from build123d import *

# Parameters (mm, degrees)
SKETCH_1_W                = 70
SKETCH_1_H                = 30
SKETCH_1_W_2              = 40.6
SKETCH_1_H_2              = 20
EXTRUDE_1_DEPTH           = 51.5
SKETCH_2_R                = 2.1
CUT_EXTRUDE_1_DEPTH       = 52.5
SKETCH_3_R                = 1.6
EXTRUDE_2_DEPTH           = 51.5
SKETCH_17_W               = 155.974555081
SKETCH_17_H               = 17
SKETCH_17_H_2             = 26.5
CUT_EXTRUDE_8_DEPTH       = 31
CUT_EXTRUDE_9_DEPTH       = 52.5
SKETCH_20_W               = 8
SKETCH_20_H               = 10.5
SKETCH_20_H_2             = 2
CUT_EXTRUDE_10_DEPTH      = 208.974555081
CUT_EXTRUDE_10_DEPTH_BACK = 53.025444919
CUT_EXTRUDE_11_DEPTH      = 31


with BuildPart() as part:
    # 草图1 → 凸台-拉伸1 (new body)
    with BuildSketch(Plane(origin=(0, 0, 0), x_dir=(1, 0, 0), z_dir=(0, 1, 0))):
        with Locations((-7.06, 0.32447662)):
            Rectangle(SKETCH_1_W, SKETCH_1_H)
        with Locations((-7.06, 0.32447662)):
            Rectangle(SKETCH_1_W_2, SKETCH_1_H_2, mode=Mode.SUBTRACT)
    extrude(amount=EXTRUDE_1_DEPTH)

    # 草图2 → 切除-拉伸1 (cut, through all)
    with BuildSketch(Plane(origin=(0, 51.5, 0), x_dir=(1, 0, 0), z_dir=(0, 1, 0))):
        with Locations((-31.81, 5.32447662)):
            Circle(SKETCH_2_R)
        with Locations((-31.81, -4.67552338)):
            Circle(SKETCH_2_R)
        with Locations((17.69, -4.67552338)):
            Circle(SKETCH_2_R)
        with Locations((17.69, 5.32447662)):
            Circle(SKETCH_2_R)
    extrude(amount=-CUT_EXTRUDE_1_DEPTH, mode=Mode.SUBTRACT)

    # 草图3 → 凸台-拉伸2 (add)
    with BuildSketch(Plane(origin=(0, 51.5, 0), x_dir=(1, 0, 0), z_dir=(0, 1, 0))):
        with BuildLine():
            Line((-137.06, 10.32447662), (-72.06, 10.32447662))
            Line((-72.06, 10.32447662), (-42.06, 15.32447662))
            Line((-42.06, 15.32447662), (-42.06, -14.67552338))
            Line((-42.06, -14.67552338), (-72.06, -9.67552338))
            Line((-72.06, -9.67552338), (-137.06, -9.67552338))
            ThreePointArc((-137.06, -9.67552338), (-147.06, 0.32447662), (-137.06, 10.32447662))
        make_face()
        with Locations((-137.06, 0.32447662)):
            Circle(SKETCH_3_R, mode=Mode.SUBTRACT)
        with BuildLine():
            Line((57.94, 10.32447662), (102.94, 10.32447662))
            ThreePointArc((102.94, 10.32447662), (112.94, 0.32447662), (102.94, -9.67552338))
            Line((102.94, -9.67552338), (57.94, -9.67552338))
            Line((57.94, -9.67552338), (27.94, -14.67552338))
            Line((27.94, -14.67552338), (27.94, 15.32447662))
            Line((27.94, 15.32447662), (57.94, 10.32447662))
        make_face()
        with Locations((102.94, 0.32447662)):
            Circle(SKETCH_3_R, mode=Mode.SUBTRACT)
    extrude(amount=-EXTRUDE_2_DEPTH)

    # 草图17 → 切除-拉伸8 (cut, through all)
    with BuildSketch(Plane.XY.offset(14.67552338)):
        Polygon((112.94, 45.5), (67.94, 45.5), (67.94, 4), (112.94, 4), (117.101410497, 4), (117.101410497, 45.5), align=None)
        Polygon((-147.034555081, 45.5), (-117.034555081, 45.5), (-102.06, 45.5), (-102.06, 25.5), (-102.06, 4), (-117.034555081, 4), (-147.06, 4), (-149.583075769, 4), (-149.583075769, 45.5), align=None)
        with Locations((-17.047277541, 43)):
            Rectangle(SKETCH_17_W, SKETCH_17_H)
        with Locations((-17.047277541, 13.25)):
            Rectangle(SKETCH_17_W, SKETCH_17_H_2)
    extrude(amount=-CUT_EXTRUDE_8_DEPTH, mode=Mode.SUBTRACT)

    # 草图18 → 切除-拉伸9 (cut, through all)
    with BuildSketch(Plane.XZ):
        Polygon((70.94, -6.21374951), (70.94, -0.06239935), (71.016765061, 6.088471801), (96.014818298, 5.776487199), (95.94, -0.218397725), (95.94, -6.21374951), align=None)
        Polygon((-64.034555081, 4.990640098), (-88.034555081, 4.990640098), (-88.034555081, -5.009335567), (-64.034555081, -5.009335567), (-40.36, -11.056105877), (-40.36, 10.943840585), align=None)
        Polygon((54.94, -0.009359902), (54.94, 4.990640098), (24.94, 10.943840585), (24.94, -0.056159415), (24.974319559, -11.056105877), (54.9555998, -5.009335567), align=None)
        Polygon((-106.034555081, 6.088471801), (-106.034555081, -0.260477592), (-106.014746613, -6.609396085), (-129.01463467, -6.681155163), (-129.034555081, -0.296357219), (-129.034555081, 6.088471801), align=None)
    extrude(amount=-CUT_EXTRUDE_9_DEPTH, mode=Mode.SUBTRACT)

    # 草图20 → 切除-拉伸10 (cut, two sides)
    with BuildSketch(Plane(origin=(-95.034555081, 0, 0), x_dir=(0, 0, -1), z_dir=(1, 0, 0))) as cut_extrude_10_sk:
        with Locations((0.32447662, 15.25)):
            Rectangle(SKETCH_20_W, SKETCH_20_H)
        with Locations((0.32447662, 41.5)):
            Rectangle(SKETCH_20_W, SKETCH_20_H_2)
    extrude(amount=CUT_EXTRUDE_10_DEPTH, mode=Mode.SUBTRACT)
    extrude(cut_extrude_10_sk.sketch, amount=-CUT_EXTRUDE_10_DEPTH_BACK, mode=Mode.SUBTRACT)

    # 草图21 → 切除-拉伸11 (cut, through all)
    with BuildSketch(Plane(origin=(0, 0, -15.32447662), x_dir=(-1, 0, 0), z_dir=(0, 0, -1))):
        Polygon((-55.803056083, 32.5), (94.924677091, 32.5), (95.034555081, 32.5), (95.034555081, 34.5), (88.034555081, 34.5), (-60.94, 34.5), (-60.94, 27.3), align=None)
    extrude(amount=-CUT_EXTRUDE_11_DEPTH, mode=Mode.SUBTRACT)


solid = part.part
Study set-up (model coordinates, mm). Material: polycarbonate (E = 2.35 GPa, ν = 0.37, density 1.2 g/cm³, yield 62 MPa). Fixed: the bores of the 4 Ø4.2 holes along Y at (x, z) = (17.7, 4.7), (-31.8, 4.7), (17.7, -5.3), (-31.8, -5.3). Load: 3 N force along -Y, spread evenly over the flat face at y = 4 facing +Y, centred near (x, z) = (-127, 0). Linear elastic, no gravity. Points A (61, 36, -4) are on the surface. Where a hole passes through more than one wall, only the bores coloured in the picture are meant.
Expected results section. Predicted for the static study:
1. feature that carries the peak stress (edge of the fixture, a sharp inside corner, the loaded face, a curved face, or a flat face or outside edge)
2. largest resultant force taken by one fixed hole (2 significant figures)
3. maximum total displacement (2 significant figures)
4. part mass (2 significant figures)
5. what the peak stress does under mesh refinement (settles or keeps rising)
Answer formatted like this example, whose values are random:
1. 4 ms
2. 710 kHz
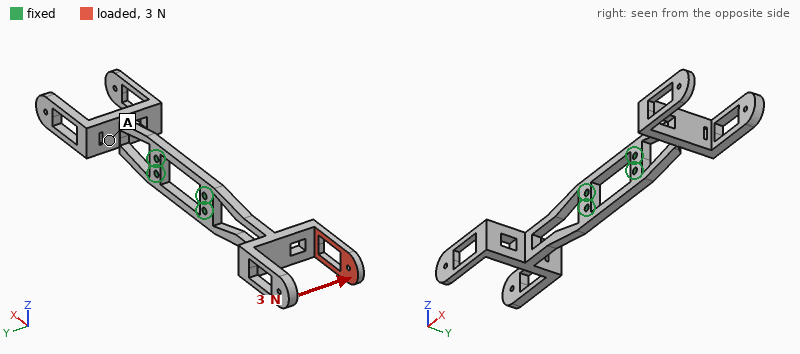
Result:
1. a sharp inside corner
2. 1.9 N
3. 3.0 mm
4. 44 g
5. keeps rising
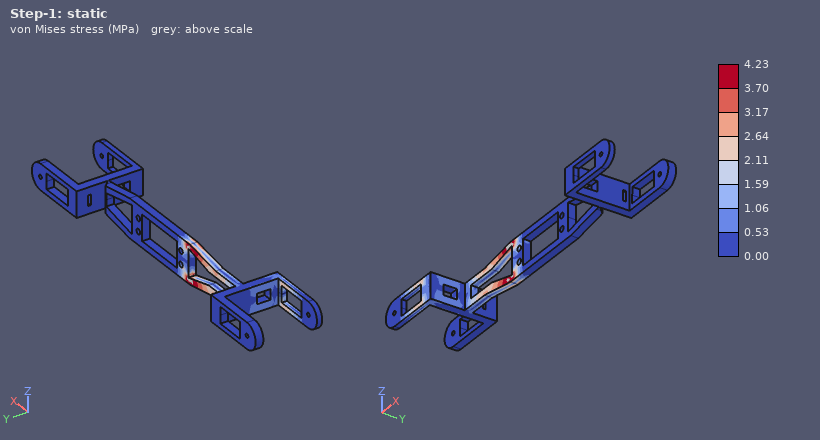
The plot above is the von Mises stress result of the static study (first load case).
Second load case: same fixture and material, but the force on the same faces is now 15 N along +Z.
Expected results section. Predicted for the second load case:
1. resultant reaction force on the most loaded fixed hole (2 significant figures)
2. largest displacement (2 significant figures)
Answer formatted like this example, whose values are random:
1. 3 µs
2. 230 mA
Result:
1. 72 N
2. 3.0 mm
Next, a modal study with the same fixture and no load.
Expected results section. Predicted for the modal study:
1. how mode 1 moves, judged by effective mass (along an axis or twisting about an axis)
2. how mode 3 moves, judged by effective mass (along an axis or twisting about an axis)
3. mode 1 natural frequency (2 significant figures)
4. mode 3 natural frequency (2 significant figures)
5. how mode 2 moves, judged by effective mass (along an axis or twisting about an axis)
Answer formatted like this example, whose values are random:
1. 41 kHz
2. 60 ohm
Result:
1. along Y
2. twisting about X
3. 60 Hz
4. 160 Hz
5. along Y
